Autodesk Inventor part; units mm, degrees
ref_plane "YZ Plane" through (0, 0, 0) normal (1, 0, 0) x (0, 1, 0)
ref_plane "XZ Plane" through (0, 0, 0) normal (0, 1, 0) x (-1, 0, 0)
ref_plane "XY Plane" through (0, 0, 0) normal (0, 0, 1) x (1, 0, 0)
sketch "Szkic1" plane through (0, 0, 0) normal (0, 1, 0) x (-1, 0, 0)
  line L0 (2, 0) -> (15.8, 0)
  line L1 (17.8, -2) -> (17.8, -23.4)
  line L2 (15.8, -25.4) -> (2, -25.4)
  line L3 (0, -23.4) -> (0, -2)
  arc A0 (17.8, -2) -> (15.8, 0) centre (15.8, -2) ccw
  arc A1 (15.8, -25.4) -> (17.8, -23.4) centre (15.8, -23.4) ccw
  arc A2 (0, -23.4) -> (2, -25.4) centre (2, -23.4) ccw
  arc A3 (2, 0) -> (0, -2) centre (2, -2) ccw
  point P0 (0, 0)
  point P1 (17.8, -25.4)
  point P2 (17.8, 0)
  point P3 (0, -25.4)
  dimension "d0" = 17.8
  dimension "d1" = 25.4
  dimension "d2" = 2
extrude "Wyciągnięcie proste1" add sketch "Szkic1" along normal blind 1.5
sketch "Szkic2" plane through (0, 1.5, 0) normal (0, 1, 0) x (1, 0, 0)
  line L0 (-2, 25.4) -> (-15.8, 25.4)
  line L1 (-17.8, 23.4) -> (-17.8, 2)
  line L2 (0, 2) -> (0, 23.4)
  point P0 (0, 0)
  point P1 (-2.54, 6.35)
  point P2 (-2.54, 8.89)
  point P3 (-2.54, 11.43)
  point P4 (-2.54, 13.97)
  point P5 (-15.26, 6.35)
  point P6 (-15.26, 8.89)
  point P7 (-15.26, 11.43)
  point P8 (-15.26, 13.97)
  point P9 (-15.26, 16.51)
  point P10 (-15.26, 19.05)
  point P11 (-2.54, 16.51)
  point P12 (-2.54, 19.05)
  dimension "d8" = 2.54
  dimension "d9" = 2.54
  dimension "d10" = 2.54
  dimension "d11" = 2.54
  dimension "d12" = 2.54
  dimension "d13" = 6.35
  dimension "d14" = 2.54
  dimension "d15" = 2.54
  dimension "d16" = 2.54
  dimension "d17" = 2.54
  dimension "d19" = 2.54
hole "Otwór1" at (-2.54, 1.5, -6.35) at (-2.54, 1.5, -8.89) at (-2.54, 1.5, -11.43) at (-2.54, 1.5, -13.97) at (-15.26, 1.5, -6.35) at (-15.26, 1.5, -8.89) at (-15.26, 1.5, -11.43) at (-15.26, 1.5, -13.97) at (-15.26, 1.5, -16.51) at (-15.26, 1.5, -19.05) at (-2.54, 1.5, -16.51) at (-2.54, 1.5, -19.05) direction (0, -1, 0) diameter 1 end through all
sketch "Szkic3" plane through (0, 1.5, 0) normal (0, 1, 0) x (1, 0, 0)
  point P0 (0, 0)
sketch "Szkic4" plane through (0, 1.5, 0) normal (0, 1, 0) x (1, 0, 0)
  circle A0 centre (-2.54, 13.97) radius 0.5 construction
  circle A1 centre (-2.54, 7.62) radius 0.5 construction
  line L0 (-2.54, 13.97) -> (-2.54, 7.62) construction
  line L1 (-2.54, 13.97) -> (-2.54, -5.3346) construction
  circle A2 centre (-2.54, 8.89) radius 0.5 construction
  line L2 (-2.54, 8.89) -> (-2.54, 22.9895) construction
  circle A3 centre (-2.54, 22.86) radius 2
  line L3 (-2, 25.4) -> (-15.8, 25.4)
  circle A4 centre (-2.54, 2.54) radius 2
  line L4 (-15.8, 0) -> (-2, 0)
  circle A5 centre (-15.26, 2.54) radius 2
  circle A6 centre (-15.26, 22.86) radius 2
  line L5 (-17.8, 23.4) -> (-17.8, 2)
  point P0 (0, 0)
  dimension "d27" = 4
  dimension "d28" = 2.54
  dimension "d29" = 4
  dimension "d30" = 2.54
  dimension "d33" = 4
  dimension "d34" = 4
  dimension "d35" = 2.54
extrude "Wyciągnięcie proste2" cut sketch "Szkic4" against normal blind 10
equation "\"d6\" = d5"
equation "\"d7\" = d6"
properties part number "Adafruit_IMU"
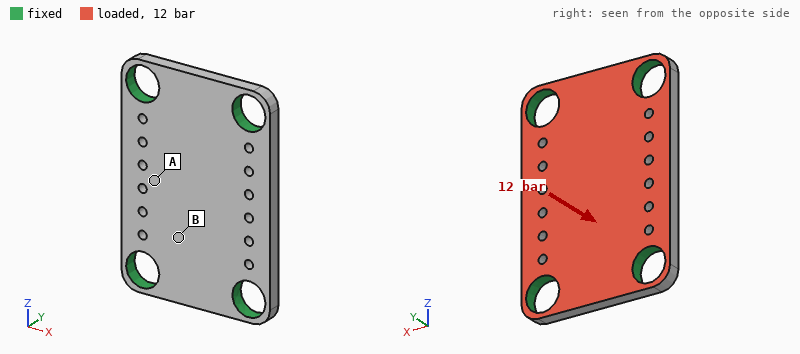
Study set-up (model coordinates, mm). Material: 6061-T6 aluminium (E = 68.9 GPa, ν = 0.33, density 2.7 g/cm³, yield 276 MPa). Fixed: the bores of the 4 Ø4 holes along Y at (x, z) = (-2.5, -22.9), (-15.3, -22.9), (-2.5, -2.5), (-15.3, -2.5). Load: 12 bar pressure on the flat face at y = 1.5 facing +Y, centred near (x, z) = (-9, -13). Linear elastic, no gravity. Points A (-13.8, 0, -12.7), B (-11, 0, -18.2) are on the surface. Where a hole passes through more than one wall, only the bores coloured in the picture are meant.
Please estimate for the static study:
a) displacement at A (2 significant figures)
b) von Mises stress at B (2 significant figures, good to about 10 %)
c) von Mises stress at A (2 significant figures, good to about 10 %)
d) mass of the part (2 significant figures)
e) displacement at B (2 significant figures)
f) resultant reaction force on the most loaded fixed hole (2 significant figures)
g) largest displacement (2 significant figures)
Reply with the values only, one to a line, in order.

18 µm
13 MPa
40 MPa
1.6 g
10 µm
120 N
19 µm
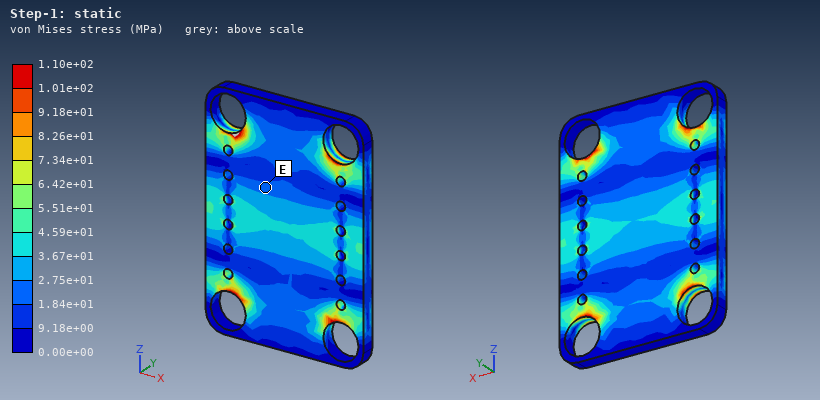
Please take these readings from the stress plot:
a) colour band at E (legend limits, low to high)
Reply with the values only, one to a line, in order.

1.84e+01 to 2.75e+01 MPa
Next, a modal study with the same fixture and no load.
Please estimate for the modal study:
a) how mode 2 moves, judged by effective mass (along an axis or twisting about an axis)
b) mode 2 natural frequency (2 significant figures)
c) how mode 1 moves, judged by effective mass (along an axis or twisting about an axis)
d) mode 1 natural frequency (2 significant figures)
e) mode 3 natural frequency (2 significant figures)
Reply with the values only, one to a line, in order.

twisting about Z
30 kHz
along Y
23 kHz
42 kHz
